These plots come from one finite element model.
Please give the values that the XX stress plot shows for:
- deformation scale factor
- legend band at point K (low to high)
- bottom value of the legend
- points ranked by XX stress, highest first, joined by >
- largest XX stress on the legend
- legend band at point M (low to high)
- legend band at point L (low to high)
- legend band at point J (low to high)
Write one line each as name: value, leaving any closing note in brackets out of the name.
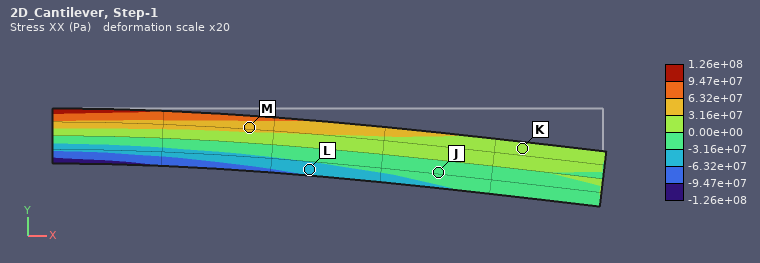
deformation scale factor: 20
legend band at point K: 0.00e+00 to 3.16e+07 Pa
bottom value of the legend: -1.26e+08 Pa
points ranked by XX stress, highest first, joined by >: M > K > J > L
largest XX stress on the legend: 1.26e+08 Pa
legend band at point M: 3.16e+07 to 6.32e+07 Pa
legend band at point L: -6.32e+07 to -3.16e+07 Pa
legend band at point J: -3.16e+07 to 0.00e+00 Pa
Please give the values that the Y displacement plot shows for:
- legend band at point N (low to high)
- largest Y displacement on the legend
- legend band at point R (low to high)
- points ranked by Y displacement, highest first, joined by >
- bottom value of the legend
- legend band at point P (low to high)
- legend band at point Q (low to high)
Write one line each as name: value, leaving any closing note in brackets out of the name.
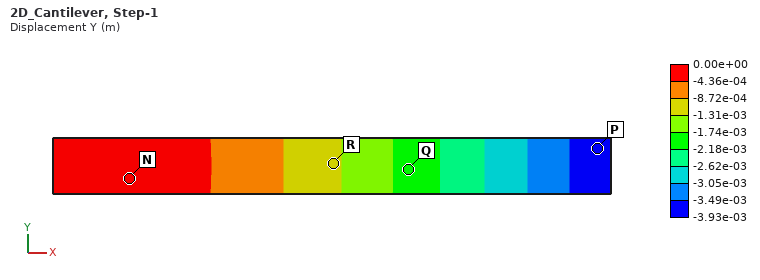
legend band at point N: -4.36e-04 to 0.00e+00 m
largest Y displacement on the legend: 0.00e+00 m
legend band at point R: -1.31e-03 to -8.72e-04 m
points ranked by Y displacement, highest first, joined by >: N > R > Q > P
bottom value of the legend: -3.93e-03 m
legend band at point P: -3.93e-03 to -3.49e-03 m
legend band at point Q: -2.18e-03 to -1.74e-03 m
